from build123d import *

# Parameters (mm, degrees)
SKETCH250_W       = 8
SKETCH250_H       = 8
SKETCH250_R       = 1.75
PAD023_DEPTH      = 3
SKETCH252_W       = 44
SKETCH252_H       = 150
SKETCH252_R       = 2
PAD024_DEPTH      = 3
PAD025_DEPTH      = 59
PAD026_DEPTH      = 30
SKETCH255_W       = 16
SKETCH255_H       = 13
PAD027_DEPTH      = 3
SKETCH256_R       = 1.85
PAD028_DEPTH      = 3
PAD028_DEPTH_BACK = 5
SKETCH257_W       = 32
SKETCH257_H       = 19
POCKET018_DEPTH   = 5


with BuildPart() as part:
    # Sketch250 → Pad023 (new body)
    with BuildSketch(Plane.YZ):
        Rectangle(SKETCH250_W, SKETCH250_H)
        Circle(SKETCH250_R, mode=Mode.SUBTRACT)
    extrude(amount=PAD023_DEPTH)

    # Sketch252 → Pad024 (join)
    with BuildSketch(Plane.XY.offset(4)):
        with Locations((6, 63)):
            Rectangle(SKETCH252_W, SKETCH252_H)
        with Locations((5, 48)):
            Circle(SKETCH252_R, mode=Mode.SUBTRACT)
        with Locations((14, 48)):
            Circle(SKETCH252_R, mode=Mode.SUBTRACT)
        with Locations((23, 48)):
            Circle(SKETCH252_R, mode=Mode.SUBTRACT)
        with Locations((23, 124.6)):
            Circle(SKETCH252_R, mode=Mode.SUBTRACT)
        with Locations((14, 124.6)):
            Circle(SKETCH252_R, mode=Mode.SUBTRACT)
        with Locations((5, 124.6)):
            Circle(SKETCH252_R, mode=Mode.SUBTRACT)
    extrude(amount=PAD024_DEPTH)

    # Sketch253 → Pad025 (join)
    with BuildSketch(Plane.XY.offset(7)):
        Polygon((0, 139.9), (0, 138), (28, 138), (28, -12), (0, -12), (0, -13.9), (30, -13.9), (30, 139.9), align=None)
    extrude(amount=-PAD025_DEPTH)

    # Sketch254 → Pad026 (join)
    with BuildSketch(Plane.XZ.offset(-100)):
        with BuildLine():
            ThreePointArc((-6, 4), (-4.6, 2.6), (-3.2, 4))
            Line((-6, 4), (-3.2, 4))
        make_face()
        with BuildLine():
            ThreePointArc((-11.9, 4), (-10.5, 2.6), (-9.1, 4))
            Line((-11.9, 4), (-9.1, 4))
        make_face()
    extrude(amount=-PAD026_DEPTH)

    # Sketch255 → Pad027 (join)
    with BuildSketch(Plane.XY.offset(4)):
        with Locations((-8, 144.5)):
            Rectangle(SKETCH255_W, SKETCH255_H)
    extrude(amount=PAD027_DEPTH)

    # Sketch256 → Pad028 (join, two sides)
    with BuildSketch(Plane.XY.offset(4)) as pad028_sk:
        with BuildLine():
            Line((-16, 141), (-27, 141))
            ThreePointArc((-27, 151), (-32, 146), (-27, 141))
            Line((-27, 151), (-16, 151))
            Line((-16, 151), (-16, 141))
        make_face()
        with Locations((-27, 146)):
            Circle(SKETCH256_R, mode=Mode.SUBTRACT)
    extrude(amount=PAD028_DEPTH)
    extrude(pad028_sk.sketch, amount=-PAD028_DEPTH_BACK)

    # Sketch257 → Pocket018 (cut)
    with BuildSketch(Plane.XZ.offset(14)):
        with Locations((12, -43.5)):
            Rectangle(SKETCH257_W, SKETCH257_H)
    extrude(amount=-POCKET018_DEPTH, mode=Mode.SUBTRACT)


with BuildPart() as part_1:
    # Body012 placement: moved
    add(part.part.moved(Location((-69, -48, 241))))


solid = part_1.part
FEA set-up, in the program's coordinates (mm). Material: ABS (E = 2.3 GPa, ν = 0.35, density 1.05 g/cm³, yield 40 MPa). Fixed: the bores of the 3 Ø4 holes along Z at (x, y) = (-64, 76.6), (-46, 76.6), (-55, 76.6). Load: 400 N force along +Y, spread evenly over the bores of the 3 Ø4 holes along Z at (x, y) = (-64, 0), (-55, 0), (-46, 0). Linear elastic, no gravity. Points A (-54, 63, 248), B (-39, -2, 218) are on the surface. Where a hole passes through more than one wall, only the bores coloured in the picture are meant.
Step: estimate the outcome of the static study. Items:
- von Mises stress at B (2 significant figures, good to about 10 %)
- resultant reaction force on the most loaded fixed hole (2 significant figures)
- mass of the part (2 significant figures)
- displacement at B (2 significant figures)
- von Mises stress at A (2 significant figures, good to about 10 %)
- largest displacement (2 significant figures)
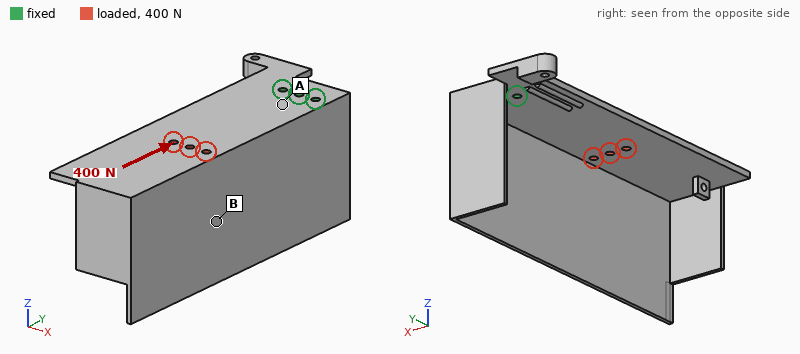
0.53 MPa
160 N
47 g
0.10 mm
3.7 MPa
0.29 mm
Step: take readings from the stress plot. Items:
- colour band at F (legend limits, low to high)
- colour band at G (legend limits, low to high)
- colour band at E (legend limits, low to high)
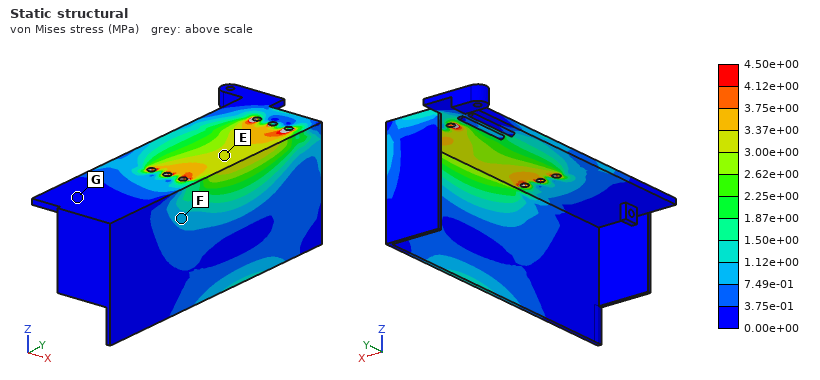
7.49e-01 to 1.12e+00 MPa
0.00e+00 to 3.75e-01 MPa
3.00e+00 to 3.37e+00 MPa
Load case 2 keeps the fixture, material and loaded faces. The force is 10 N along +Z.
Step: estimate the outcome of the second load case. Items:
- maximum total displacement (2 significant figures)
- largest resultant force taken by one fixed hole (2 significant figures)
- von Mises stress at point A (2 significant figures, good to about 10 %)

2.2 mm
6.8 N
2.2 MPa
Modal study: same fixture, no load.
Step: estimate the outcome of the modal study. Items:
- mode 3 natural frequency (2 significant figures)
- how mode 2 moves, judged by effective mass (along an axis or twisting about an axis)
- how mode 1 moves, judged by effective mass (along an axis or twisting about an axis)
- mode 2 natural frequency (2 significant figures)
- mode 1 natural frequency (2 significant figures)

240 Hz
along X
along Z
92 Hz
69 Hz
